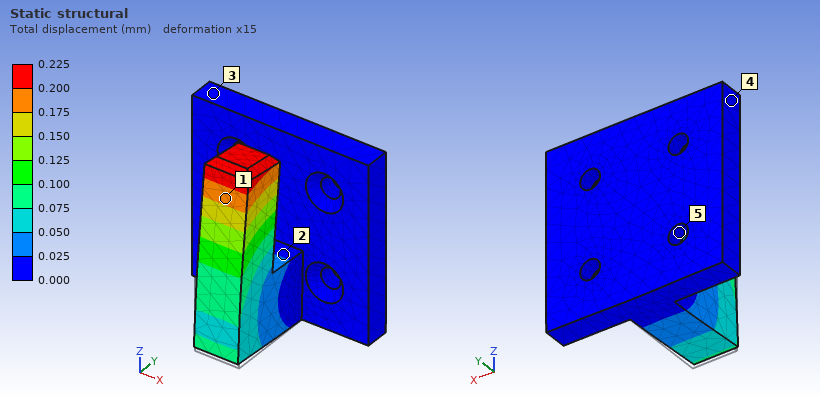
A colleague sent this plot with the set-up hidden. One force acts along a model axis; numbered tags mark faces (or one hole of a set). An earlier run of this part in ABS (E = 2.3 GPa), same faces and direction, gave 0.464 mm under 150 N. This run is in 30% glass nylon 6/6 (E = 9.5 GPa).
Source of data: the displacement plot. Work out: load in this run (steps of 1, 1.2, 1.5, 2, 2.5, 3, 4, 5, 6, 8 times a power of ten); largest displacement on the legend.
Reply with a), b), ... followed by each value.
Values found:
a) 300 N
b) 0.225 mm
